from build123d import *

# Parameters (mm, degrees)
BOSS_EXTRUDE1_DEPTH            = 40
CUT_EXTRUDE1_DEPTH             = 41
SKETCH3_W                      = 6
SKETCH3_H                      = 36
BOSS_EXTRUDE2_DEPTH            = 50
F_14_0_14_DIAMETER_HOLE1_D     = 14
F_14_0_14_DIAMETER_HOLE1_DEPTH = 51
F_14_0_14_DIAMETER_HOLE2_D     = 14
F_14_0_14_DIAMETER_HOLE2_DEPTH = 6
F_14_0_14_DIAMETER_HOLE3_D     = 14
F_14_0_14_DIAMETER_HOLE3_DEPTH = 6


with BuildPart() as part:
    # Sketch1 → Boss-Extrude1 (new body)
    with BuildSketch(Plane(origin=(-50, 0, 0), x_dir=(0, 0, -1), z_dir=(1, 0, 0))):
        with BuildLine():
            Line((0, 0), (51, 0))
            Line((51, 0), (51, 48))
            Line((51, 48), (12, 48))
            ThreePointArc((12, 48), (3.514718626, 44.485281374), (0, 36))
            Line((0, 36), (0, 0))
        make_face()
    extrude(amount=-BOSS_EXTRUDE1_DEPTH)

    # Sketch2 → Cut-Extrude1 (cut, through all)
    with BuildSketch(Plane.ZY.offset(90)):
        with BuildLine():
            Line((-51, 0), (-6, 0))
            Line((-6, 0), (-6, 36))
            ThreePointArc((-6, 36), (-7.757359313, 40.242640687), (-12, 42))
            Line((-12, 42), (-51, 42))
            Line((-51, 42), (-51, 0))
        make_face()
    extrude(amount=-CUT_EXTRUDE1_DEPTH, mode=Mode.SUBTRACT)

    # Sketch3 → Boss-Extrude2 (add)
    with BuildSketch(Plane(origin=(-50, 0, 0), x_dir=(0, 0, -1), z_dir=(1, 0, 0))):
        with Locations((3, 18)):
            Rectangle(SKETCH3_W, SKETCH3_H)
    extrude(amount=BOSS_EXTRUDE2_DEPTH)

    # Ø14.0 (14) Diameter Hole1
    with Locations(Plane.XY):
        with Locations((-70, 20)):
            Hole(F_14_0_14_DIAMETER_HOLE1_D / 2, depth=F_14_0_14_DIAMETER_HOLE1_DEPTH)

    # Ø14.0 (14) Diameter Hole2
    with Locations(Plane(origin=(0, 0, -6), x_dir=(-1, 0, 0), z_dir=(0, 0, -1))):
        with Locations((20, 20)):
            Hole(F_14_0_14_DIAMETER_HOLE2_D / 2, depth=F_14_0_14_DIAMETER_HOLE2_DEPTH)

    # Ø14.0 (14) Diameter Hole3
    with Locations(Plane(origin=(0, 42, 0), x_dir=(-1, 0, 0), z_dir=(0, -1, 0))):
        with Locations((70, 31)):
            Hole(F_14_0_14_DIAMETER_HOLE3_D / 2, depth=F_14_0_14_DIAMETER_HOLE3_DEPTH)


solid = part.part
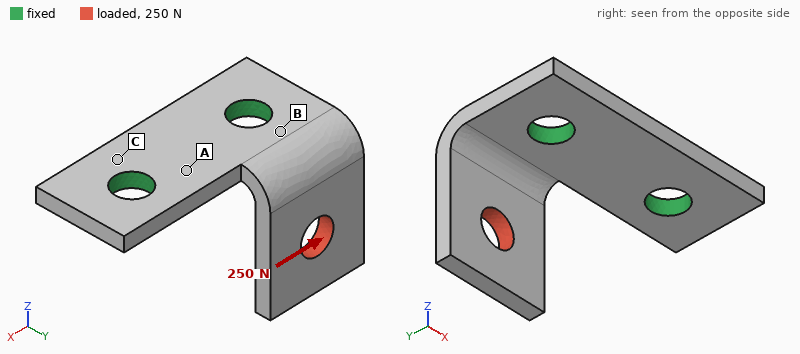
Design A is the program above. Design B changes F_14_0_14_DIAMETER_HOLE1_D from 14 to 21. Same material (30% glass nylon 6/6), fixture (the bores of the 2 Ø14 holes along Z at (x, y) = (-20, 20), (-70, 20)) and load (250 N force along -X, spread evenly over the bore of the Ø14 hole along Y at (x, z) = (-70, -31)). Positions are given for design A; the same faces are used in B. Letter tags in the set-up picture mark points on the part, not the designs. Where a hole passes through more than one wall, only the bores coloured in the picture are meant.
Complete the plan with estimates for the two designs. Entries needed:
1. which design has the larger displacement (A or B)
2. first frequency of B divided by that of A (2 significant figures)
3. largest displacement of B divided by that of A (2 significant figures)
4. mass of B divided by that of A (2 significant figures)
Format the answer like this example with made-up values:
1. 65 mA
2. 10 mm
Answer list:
1. A
2. 1.1
3. 0.74
4. 0.96
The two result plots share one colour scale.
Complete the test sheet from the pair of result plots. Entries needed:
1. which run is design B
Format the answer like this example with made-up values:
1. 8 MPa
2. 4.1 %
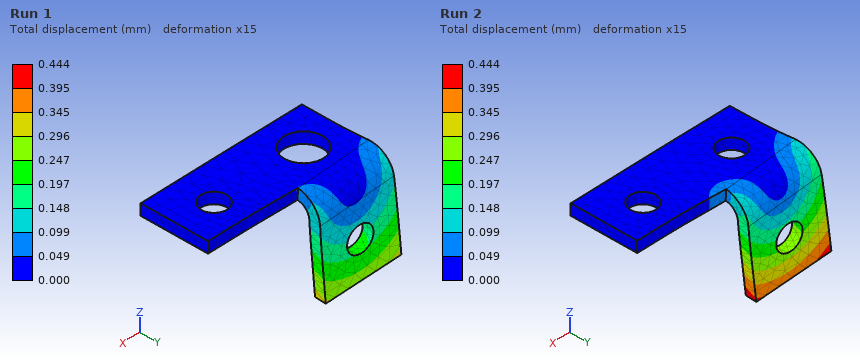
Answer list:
1. Run 1
